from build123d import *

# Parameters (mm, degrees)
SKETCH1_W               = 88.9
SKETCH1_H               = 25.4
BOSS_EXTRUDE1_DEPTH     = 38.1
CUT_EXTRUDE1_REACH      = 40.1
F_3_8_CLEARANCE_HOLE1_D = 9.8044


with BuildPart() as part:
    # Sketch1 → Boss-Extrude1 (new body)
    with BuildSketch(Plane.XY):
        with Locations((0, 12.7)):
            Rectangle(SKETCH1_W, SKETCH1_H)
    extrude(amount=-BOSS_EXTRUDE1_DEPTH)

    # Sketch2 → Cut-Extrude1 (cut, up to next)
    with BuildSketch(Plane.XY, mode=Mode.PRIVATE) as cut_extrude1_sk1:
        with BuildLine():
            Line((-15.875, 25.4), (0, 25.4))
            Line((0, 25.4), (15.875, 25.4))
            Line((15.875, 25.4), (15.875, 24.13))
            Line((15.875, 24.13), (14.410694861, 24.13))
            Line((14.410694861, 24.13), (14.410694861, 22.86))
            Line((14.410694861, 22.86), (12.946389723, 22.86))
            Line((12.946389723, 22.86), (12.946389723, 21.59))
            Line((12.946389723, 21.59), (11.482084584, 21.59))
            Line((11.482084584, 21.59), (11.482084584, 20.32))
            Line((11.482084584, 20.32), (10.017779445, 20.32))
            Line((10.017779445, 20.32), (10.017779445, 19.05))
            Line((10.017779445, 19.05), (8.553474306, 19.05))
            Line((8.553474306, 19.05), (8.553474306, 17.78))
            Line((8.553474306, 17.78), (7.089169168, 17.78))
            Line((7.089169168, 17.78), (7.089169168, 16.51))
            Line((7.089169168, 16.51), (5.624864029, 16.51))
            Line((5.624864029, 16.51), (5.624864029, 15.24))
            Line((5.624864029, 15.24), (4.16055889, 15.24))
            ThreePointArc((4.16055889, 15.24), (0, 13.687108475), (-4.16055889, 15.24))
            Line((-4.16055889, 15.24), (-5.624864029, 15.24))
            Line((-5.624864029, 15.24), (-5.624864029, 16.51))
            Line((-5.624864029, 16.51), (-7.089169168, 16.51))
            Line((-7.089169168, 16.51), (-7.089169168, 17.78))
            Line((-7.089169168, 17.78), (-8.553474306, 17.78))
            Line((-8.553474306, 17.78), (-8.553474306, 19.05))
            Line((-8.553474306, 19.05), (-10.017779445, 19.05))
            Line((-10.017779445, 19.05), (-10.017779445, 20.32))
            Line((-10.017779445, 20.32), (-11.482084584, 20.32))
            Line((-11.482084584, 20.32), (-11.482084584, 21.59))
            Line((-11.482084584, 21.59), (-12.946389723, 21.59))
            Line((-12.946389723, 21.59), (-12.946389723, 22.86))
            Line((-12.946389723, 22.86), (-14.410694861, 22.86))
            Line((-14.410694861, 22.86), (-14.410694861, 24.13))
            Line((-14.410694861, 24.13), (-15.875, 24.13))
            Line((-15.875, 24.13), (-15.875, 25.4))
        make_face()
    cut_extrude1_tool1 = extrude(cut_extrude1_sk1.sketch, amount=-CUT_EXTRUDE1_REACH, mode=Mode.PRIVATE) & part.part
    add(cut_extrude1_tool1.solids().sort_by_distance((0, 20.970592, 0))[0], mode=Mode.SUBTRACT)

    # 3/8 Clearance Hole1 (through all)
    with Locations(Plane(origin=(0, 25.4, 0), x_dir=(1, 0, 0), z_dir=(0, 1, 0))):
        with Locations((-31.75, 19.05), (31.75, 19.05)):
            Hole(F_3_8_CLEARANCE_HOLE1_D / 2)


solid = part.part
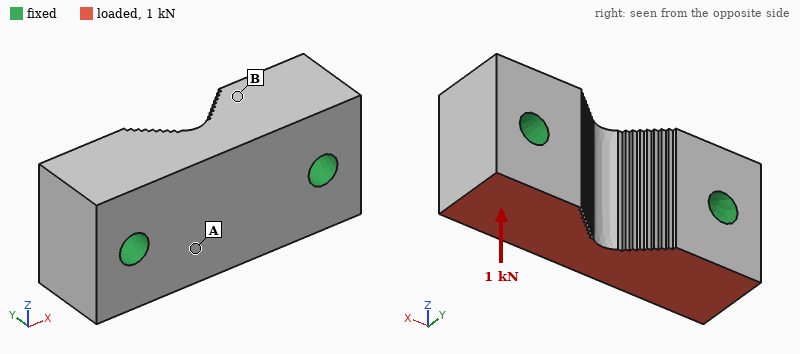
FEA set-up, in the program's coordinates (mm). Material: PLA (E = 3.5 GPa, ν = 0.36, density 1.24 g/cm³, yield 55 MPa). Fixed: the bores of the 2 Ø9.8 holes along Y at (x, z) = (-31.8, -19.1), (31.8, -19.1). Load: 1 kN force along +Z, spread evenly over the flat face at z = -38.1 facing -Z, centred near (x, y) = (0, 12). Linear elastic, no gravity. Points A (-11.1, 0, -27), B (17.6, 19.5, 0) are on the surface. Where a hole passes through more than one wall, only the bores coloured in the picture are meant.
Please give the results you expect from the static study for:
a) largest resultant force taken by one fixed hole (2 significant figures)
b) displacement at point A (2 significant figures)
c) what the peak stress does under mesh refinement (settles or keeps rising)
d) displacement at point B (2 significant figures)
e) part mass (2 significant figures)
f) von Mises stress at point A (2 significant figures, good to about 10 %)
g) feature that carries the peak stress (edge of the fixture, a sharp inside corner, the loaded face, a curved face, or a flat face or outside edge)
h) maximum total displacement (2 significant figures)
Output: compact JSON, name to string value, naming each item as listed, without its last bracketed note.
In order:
{"largest resultant force taken by one fixed hole": "500 N", "displacement at point A": "7.7 µm", "what the peak stress does under mesh refinement": "keeps rising", "displacement at point B": "4.5 µm", "part mass": "91 g", "von Mises stress at point A": "0.53 MPa", "feature that carries the peak stress": "edge of the fixture", "maximum total displacement": "11 µm"}
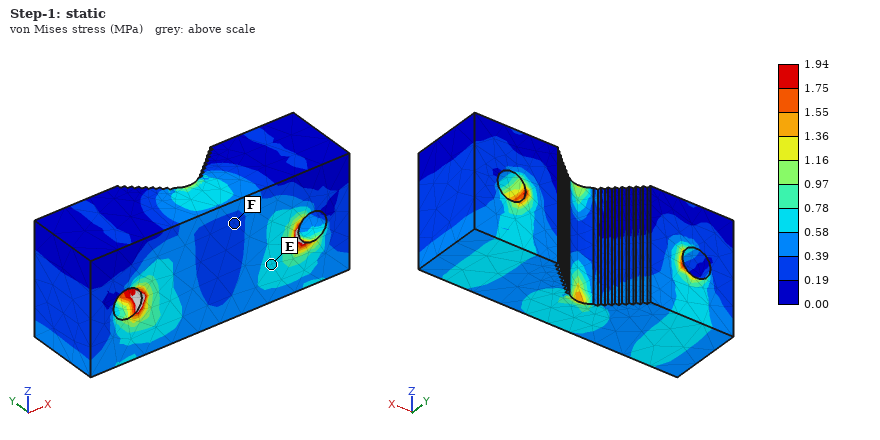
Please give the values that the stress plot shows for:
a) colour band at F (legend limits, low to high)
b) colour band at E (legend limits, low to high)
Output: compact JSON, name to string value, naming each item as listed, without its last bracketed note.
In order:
{"colour band at F": "0.19 to 0.39 MPa", "colour band at E": "0.58 to 0.78 MPa"}
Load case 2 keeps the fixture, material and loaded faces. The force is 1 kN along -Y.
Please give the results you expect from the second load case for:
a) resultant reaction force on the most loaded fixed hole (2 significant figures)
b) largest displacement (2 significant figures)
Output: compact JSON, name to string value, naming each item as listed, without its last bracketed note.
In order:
{"resultant reaction force on the most loaded fixed hole": "500 N", "largest displacement": "33 µm"}
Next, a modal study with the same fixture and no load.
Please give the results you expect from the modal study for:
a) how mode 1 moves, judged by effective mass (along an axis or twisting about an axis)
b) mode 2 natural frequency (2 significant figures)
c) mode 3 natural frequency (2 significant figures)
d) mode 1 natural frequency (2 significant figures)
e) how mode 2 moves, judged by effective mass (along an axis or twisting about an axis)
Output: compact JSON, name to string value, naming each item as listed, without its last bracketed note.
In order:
{"how mode 1 moves, judged by effective mass": "along Z", "mode 2 natural frequency": "6300 Hz", "mode 3 natural frequency": "7600 Hz", "mode 1 natural frequency": "5900 Hz", "how mode 2 moves, judged by effective mass": "along Y"}
